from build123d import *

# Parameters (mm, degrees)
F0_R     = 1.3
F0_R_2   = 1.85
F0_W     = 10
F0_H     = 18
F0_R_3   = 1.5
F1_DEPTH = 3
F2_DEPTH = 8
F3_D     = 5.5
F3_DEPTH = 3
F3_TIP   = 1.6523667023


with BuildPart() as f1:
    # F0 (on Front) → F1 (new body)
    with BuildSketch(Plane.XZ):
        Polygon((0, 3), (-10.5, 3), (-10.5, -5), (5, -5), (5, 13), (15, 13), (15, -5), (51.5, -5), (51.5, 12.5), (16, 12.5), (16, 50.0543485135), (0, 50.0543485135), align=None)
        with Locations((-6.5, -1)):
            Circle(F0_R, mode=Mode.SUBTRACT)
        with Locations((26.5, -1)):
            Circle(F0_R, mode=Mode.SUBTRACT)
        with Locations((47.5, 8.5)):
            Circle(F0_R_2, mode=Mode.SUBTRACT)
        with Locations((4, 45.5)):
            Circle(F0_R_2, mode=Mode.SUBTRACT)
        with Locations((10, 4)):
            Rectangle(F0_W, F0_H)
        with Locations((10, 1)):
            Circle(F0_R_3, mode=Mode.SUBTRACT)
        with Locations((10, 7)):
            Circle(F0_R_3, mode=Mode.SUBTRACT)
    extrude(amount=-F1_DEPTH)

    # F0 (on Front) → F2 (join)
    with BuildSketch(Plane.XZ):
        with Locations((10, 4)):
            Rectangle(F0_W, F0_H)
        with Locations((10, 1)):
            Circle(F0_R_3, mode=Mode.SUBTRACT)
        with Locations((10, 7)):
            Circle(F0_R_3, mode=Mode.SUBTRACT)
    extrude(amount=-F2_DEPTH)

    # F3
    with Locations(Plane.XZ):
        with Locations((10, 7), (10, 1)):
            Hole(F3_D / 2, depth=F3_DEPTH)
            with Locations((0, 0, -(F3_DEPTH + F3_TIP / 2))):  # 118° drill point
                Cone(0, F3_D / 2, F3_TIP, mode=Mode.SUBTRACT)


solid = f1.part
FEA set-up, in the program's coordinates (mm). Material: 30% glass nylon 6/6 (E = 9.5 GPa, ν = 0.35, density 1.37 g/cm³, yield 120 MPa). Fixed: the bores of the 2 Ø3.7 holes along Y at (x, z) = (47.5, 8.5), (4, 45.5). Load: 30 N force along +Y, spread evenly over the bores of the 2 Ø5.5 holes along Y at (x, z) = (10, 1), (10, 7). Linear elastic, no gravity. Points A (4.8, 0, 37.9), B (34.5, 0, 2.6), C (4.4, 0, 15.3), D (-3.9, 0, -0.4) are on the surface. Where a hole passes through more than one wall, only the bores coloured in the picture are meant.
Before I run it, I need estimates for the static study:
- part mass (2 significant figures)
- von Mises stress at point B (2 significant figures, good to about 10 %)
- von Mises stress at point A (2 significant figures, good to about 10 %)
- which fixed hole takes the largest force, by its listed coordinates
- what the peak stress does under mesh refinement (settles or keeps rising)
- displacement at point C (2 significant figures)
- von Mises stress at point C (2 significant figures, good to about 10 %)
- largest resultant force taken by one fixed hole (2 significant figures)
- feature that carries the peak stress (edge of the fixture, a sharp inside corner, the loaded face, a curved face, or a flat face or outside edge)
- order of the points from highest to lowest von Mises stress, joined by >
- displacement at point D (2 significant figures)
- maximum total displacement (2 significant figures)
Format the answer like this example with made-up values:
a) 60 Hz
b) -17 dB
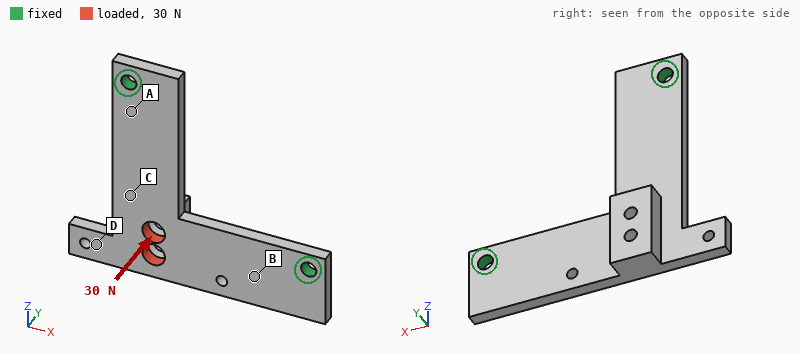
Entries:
a) 7.3 g
b) 9.4 MPa
c) 14 MPa
d) (47.5, 8.5)
e) keeps rising
f) 0.35 mm
g) 5.7 MPa
h) 17 N
i) edge of the fixture
j) A > B > C > D
k) 0.70 mm
l) 0.86 mm
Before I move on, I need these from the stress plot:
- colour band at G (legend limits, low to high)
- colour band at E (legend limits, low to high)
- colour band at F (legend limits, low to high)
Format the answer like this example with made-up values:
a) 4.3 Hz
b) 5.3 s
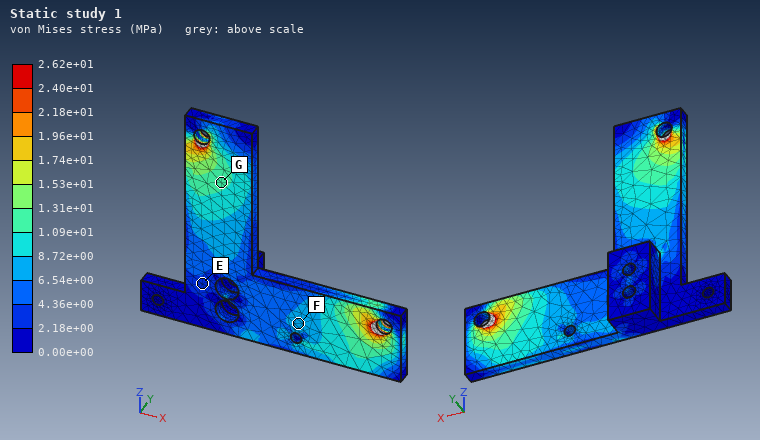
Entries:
a) 1.09e+01 to 1.31e+01 MPa
b) 2.18e+00 to 4.36e+00 MPa
c) 6.54e+00 to 8.72e+00 MPa
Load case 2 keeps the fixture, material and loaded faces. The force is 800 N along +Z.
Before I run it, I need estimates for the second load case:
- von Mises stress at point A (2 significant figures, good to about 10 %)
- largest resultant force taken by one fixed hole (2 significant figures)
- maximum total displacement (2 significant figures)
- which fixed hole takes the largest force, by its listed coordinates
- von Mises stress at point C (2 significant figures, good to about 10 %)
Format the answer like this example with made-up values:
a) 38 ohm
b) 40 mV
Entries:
a) 24 MPa
b) 760 N
c) 0.12 mm
d) (4, 45.5)
e) 16 MPa
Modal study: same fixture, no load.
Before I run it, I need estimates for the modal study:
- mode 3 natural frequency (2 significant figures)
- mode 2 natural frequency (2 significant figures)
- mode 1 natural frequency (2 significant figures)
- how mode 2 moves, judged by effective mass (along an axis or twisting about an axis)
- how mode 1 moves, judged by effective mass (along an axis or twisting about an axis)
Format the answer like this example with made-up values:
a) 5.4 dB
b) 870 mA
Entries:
a) 2900 Hz
b) 2600 Hz
c) 650 Hz
d) along Y
e) along Y
